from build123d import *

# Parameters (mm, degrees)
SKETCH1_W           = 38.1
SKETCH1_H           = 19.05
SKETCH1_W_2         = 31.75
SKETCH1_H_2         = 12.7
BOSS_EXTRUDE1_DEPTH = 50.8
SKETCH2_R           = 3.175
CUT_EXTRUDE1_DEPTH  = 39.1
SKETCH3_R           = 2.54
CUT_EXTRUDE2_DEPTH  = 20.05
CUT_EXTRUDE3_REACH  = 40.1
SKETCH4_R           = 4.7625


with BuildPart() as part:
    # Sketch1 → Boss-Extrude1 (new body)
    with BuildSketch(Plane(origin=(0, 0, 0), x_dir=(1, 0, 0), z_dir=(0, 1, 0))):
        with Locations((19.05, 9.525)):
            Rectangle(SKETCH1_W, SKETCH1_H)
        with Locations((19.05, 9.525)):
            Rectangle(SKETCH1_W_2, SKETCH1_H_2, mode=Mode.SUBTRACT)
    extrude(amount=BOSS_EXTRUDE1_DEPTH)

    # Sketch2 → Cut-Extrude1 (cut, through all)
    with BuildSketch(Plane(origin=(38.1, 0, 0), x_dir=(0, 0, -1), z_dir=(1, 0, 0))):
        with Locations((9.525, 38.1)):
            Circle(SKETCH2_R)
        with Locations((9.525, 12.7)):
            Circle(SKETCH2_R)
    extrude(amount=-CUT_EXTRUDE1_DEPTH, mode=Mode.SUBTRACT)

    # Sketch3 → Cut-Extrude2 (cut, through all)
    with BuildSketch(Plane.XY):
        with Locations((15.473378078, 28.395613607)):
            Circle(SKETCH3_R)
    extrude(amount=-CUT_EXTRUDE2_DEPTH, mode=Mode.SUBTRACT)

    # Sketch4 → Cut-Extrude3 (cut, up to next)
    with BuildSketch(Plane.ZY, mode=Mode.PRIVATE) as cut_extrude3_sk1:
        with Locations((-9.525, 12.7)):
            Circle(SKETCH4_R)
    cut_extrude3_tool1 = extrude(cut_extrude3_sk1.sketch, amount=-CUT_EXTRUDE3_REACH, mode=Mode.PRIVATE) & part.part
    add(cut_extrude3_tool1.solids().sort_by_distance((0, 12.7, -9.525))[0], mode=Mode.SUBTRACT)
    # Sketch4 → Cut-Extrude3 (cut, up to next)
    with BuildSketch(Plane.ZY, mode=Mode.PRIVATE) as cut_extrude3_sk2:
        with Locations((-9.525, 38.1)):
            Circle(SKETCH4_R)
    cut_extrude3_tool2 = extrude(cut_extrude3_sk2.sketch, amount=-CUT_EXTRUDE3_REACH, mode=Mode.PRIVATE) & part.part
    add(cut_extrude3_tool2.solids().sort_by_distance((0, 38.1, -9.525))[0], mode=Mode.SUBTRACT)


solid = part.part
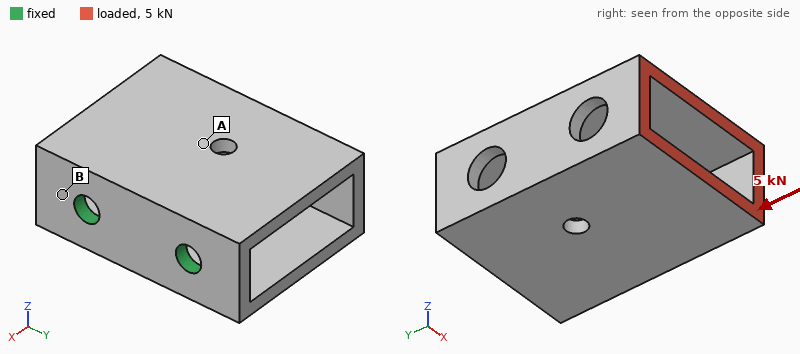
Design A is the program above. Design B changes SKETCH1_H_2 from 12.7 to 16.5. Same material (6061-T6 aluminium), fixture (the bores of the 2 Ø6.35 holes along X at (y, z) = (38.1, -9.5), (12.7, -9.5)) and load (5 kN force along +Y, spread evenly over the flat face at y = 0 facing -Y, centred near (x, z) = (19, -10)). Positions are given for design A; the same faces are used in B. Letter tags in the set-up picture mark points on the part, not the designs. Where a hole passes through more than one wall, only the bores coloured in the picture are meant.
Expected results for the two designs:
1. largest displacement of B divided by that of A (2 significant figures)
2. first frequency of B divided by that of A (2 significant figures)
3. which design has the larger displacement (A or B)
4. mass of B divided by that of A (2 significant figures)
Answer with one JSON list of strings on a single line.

["1.9", "0.51", "B", "0.61"]
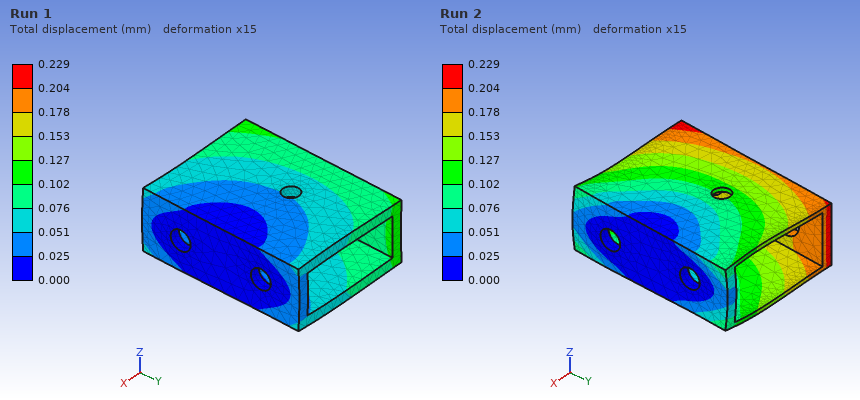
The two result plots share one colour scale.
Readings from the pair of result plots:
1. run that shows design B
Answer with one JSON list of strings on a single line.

["Run 2"]
